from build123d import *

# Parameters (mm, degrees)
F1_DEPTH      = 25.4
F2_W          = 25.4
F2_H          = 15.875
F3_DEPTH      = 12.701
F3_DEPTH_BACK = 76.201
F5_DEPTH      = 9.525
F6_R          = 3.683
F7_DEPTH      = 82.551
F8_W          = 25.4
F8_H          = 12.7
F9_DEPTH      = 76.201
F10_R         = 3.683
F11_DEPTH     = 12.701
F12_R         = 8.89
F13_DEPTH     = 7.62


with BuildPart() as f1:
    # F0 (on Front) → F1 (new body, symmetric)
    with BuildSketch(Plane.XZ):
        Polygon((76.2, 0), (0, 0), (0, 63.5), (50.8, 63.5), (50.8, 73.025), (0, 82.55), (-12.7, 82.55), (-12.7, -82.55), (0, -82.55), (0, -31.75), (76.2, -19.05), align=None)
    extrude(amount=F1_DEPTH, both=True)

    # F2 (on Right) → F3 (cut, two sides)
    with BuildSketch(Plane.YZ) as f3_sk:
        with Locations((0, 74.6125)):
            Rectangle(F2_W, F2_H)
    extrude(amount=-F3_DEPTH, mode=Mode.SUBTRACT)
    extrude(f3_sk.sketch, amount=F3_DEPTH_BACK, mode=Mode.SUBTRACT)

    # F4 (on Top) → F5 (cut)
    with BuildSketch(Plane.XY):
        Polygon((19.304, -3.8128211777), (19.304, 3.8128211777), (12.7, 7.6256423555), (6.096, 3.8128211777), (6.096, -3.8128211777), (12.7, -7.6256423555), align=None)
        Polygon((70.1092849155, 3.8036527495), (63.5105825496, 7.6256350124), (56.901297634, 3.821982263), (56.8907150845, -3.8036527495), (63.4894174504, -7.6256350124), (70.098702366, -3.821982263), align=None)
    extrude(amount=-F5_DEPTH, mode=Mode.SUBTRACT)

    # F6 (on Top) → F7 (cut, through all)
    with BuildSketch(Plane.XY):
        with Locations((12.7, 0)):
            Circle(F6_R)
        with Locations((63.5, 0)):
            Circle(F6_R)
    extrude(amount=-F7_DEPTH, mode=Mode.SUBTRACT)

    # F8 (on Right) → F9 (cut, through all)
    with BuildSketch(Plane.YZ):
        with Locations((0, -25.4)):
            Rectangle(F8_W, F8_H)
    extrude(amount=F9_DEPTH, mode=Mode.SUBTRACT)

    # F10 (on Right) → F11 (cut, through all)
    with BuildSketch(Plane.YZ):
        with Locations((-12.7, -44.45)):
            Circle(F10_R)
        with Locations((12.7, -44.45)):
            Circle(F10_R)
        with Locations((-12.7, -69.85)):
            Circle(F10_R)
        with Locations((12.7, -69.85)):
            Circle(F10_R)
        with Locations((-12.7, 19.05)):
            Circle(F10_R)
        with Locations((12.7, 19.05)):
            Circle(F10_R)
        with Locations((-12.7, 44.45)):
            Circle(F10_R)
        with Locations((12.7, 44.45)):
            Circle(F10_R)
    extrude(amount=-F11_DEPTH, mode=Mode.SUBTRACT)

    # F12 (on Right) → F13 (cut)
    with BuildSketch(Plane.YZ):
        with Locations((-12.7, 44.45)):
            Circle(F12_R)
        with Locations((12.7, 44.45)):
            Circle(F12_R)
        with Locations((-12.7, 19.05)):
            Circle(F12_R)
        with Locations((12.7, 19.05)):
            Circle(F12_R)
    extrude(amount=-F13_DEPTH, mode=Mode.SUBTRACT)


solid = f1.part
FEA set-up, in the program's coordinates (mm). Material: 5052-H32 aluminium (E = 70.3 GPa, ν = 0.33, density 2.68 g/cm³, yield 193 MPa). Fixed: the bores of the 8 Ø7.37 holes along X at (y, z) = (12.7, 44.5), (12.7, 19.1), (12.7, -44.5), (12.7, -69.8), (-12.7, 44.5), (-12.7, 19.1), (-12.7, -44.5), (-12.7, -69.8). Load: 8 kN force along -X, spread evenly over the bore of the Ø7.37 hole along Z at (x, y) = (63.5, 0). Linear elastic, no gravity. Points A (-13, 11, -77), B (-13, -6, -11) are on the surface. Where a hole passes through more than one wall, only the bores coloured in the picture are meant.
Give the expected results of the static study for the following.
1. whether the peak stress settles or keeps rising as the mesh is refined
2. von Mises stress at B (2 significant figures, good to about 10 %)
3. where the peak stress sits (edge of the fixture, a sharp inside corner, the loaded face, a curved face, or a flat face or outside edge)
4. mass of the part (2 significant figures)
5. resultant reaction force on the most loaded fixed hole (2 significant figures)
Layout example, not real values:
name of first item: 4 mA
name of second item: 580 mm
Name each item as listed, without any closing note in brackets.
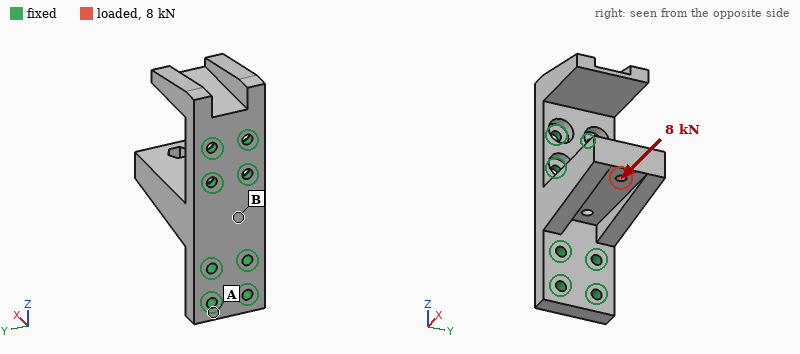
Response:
whether the peak stress settles or keeps rising as the mesh is refined: keeps rising
von Mises stress at B: 14 MPa
where the peak stress sits: edge of the fixture
mass of the part: 520 g
resultant reaction force on the most loaded fixed hole: 2.6 kN
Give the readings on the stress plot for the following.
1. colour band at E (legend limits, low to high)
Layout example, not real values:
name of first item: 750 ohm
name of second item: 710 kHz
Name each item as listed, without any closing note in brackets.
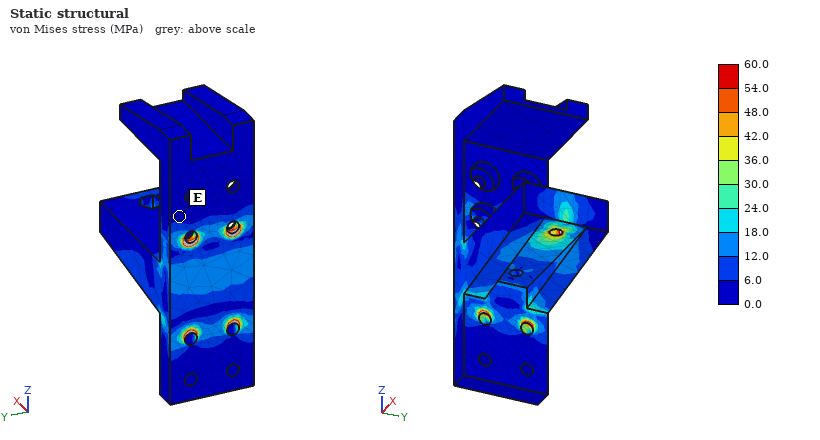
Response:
colour band at E: 0.0 to 6.0 MPa
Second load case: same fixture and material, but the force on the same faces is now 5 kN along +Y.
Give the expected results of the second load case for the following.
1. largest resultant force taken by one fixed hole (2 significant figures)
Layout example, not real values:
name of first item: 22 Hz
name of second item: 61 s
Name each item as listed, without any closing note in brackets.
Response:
largest resultant force taken by one fixed hole: 7.3 kN
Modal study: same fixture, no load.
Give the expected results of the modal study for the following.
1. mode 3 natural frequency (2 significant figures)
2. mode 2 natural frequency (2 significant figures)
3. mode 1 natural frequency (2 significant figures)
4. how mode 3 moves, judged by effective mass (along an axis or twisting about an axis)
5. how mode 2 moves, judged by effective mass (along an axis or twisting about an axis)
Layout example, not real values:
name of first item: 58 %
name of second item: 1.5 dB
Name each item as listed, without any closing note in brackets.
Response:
mode 3 natural frequency: 2700 Hz
mode 2 natural frequency: 2300 Hz
mode 1 natural frequency: 1800 Hz
how mode 3 moves, judged by effective mass: along Z
how mode 2 moves, judged by effective mass: along Y
